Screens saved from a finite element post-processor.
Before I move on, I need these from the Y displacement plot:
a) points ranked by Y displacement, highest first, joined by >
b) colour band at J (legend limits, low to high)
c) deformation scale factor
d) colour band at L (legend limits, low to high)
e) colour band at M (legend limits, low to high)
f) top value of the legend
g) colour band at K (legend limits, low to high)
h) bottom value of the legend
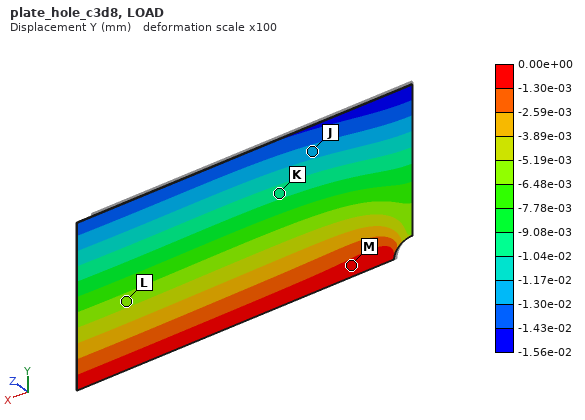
M > L > K > J
-1.30e-02 to -1.17e-02 mm
100
-6.48e-03 to -5.19e-03 mm
-1.30e-03 to 0.00e+00 mm
0.00e+00 mm
-1.04e-02 to -9.08e-03 mm
-1.56e-02 mm
